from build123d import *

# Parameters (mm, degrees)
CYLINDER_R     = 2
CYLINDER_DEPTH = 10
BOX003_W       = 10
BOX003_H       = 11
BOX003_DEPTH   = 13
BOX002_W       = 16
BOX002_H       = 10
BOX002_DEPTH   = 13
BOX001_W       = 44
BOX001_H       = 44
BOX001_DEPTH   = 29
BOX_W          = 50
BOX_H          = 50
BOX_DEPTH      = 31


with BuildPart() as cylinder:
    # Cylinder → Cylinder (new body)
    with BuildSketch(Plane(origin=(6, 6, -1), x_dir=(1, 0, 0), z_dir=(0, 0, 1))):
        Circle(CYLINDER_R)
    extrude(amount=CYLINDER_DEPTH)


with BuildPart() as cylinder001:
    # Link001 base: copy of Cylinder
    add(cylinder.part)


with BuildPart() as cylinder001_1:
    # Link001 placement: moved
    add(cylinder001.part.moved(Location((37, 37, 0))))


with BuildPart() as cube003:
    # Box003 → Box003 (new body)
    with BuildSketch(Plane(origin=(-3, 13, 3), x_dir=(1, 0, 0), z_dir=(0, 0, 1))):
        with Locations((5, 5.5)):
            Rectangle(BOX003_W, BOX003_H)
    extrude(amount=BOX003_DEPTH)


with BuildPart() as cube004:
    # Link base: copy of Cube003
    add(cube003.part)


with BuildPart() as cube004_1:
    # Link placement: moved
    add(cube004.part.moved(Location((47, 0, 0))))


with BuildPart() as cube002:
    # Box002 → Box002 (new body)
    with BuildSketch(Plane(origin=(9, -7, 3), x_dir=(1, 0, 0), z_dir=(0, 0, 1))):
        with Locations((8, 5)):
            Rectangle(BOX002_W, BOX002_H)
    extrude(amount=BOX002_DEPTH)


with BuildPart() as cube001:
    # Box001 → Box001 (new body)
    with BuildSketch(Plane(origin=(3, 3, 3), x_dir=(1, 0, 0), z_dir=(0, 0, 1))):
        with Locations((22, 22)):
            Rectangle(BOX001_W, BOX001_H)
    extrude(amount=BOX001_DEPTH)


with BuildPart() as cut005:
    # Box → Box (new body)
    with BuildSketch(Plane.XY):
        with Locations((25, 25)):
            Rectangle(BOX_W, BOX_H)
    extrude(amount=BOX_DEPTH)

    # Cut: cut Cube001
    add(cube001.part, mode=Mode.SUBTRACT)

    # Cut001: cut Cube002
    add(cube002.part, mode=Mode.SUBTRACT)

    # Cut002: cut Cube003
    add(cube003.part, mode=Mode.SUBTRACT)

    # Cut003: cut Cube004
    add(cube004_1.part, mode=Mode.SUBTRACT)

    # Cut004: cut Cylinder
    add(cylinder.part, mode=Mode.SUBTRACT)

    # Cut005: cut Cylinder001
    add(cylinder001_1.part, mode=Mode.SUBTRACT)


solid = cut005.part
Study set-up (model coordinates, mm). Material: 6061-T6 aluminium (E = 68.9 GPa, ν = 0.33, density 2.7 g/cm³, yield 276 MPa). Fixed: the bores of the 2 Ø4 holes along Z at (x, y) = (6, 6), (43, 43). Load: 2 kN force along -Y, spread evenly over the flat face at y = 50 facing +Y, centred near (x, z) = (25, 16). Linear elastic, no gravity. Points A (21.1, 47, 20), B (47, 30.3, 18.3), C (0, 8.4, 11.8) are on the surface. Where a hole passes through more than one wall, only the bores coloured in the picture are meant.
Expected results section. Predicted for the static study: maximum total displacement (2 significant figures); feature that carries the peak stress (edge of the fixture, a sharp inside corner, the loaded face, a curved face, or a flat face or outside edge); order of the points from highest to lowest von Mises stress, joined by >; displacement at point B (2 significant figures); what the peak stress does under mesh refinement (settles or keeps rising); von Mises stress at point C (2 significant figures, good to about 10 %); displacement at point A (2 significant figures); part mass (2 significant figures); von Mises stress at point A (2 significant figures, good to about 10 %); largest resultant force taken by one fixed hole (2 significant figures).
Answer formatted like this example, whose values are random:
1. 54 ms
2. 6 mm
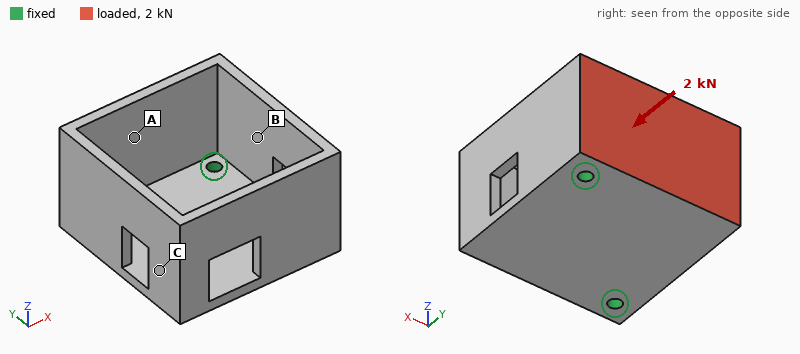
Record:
1. 0.34 mm
2. edge of the fixture
3. A > C > B
4. 0.13 mm
5. keeps rising
6. 34 MPa
7. 0.22 mm
8. 59 g
9. 55 MPa
10. 1.1 kN
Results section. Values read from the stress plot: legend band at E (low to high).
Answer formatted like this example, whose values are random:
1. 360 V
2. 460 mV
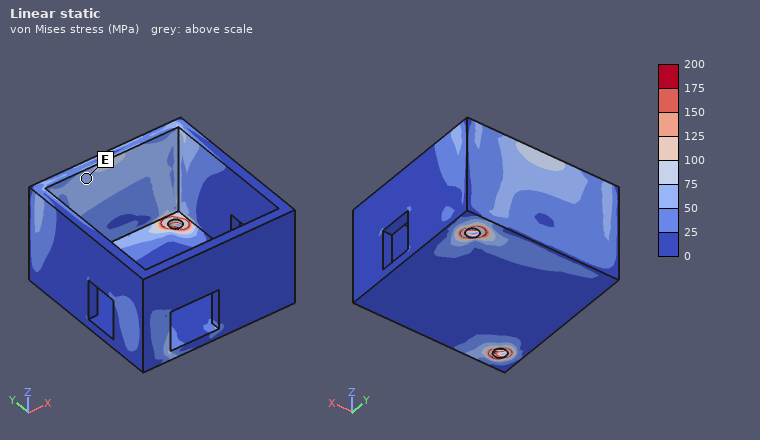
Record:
1. 50 to 75 MPa
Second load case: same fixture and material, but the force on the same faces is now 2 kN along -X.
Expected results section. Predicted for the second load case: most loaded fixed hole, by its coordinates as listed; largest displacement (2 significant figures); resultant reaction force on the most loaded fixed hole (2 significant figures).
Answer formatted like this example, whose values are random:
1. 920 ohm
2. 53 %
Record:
1. (43, 43)
2. 0.41 mm
3. 2.0 kN
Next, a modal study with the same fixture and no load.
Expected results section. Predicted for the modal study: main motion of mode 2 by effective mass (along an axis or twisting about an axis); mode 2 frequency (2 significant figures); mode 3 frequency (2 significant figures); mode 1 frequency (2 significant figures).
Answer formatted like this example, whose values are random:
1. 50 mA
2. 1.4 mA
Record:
1. along Z
2. 2300 Hz
3. 5100 Hz
4. 1700 Hz
